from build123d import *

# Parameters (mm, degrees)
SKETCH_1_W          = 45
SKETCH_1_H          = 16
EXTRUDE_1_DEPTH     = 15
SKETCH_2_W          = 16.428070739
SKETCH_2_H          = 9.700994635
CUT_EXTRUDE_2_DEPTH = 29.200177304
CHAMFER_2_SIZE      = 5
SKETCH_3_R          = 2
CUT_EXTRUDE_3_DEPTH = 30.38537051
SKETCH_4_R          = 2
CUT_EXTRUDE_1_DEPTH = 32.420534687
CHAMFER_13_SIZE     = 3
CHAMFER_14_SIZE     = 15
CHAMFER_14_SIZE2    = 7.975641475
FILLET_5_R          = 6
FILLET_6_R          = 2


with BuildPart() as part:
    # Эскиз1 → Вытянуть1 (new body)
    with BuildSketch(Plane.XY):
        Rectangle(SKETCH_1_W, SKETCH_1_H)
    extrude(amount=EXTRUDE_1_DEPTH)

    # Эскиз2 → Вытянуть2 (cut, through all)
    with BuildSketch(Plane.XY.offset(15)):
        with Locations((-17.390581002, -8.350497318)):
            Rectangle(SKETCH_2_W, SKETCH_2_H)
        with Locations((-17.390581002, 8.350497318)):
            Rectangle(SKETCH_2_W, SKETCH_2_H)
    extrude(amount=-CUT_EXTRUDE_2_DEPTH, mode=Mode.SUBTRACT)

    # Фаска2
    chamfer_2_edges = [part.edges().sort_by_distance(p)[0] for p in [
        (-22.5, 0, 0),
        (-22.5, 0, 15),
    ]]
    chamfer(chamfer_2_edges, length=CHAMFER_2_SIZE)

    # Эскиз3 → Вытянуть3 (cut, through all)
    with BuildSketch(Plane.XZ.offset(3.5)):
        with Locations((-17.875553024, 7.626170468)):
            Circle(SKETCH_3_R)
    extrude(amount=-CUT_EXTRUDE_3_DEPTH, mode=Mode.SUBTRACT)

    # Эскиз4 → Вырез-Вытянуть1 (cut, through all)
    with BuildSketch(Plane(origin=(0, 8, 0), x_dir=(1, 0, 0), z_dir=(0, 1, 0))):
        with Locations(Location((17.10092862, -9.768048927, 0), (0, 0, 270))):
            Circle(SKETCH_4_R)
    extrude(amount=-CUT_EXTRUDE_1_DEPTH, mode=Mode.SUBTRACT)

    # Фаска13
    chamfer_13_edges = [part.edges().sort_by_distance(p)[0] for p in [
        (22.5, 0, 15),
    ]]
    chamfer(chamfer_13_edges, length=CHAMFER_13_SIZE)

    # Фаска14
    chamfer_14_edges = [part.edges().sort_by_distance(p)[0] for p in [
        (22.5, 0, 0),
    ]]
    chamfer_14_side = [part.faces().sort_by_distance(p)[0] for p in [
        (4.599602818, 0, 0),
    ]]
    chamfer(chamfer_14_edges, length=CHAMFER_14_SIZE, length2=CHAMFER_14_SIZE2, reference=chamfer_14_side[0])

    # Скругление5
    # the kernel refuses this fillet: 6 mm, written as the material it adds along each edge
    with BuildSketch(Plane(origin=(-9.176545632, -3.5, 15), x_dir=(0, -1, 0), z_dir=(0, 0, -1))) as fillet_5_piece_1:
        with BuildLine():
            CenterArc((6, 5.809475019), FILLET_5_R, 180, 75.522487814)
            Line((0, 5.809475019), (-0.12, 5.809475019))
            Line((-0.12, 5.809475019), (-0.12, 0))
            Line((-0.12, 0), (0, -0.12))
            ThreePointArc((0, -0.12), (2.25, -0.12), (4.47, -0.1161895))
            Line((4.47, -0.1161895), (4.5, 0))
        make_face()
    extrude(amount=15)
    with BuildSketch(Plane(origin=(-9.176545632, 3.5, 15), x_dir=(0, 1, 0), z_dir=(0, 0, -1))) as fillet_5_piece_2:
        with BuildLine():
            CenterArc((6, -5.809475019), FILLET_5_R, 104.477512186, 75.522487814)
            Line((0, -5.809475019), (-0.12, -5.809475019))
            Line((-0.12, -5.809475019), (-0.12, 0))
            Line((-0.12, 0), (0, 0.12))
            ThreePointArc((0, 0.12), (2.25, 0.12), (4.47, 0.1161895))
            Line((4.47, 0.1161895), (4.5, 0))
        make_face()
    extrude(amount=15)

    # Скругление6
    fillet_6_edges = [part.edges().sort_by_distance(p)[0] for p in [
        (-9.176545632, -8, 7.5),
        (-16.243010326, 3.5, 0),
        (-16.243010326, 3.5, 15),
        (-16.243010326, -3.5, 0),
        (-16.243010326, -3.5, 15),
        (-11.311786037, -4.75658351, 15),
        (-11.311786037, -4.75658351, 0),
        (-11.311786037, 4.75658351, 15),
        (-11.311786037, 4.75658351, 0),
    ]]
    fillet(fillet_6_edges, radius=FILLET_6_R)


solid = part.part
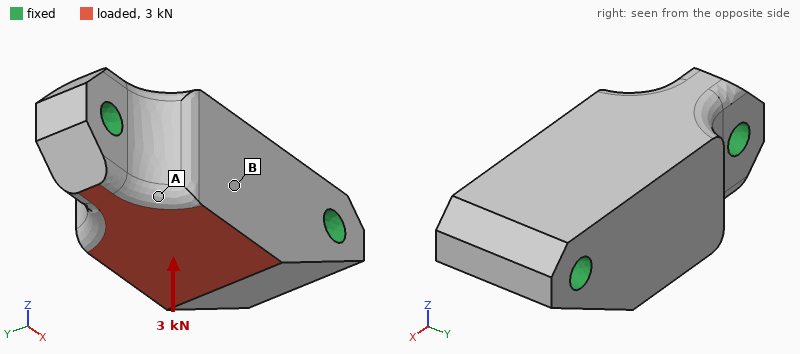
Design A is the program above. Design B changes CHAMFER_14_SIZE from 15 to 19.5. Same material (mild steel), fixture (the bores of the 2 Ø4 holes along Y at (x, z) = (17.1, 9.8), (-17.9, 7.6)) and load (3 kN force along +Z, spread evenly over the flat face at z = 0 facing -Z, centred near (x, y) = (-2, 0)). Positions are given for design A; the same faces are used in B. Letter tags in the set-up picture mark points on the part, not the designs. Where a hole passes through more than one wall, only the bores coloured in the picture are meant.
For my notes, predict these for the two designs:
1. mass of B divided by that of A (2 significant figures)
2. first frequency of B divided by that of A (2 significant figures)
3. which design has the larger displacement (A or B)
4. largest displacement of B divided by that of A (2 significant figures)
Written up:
0.96
1.00
B
1.1
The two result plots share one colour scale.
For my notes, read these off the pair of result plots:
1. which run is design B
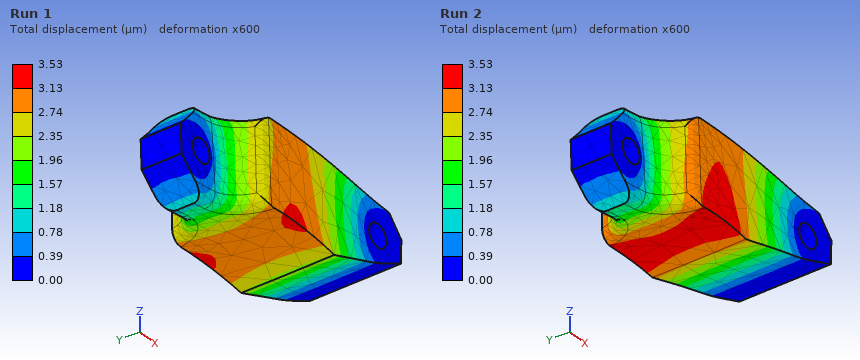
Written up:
Run 2
